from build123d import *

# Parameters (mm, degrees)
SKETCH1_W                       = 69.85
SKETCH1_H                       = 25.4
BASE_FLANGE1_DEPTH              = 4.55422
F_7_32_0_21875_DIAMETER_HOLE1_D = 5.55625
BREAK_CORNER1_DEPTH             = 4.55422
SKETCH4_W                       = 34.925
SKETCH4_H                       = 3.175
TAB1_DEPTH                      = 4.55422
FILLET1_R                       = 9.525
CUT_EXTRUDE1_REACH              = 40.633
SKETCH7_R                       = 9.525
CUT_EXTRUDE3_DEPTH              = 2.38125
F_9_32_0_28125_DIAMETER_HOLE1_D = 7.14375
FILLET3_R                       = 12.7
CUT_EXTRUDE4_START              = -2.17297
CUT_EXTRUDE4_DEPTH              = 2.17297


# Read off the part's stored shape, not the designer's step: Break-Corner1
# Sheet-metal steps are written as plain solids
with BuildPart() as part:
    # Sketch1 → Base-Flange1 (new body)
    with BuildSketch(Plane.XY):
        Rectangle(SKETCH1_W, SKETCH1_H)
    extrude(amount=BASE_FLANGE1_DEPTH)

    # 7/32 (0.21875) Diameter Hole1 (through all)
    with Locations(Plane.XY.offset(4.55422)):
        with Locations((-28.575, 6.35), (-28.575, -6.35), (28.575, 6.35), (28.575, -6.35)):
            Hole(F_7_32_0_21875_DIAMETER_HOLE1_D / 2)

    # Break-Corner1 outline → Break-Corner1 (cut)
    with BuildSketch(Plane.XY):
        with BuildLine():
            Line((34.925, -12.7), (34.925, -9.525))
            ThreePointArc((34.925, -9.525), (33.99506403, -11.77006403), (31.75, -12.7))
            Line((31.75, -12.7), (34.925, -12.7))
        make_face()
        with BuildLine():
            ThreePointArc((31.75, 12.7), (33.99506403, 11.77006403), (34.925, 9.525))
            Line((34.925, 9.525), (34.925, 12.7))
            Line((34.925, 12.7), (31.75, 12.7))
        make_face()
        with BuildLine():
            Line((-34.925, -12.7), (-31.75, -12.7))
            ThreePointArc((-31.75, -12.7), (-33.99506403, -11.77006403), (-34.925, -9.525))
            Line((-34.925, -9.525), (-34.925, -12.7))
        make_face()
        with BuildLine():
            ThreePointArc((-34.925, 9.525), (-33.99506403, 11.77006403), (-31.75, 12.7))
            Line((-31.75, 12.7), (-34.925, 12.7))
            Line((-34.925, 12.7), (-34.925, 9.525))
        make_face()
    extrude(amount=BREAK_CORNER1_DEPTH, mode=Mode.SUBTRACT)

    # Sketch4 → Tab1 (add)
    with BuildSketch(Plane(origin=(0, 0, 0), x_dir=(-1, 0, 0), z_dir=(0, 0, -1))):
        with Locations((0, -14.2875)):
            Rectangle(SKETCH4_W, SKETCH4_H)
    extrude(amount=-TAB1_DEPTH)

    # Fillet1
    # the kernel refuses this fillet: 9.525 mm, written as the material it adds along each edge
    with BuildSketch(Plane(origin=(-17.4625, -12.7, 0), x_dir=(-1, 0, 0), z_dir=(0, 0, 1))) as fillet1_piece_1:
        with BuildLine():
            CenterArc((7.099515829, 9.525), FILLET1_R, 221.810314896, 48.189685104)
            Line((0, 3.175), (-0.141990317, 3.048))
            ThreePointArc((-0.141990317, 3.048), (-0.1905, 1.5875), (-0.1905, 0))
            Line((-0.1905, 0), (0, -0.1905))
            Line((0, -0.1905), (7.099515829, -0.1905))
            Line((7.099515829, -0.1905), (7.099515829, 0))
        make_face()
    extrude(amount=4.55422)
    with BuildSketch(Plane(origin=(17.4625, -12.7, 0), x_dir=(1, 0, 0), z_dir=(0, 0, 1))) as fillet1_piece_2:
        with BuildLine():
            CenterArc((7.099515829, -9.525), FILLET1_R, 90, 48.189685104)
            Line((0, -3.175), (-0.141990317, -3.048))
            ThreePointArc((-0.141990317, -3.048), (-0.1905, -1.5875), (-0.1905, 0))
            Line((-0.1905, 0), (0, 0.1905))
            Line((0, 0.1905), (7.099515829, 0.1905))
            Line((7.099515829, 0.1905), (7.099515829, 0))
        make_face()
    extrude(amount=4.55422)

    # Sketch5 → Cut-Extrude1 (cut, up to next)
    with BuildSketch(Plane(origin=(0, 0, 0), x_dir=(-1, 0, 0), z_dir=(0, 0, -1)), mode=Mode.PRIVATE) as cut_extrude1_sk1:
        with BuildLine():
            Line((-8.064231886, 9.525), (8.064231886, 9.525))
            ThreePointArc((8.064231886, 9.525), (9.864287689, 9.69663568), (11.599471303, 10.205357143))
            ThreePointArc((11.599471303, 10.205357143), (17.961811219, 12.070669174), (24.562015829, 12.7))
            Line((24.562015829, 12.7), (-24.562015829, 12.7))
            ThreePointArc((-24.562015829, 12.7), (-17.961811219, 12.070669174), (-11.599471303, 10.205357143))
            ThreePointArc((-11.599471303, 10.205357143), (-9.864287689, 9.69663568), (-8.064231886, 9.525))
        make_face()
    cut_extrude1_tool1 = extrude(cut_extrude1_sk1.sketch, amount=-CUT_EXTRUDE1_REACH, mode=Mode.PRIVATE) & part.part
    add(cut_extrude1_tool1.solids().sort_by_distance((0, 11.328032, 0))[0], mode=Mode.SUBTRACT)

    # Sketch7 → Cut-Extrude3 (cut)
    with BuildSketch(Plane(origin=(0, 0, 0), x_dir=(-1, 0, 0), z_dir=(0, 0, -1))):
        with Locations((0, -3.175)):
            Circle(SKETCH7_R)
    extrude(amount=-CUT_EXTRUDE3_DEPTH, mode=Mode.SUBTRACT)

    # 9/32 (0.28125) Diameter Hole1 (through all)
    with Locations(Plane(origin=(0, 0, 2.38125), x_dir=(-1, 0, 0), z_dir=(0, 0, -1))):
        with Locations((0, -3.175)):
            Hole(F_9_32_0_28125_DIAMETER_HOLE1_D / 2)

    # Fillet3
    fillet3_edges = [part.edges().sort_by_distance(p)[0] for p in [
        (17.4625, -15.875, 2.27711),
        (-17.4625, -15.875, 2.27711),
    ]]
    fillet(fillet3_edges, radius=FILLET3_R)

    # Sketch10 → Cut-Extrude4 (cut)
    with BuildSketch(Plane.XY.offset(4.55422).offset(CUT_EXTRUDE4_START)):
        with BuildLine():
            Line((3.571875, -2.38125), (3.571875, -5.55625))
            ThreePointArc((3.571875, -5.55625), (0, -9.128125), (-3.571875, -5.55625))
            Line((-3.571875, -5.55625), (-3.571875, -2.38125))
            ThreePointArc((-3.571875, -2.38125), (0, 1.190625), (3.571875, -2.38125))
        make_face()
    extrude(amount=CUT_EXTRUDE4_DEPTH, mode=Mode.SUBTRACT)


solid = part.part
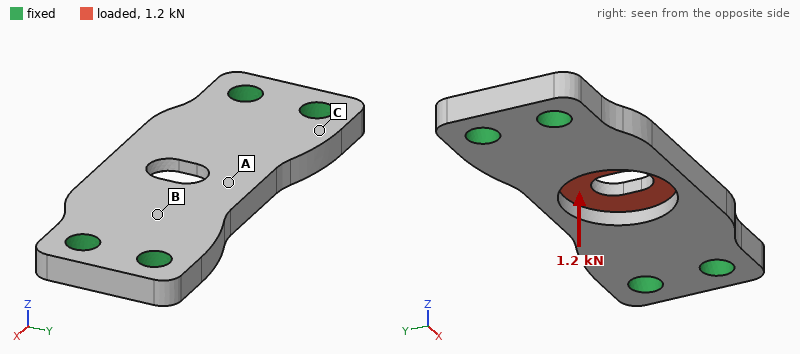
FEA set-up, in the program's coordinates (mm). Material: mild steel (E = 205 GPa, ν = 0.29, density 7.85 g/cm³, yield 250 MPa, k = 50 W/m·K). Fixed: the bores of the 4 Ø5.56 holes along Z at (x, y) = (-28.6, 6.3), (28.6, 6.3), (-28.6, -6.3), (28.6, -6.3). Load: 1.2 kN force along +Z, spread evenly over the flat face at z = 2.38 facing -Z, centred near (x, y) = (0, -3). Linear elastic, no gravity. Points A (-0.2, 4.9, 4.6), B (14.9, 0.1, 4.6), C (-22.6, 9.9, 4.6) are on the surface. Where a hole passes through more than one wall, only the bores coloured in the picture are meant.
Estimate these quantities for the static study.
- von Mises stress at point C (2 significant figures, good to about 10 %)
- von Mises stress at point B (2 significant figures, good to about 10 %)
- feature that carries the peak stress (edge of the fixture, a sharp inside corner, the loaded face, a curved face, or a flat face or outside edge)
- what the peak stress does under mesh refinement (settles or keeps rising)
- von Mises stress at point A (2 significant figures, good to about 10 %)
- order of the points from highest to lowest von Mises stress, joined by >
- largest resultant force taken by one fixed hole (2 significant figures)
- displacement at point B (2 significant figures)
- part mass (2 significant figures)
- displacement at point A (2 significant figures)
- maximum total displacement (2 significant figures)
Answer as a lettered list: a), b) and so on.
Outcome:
a) 57 MPa
b) 23 MPa
c) edge of the fixture
d) keeps rising
e) 110 MPa
f) A > C > B
g) 490 N
h) 13 µm
i) 54 g
j) 31 µm
k) 36 µm
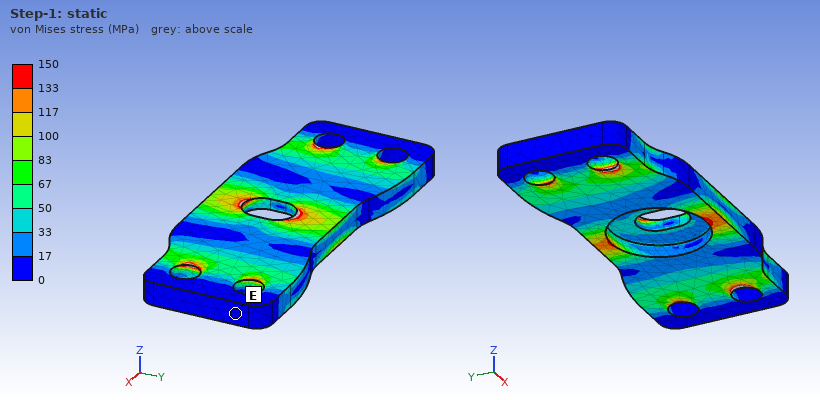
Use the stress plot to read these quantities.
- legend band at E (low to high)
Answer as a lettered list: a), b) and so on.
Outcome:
a) 0 to 17 MPa
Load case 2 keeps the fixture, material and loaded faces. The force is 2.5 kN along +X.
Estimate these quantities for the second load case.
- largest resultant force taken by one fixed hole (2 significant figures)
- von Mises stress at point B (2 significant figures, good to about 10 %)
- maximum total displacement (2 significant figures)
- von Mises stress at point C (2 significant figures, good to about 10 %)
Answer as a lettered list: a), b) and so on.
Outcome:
a) 730 N
b) 18 MPa
c) 2.4 µm
d) 8.8 MPa
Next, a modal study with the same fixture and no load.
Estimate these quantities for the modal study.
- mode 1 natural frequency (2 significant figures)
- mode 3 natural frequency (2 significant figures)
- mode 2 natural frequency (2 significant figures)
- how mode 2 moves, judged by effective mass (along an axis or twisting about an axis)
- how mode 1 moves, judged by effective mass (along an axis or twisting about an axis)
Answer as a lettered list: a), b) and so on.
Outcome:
a) 8100 Hz
b) 18 kHz
c) 12 kHz
d) twisting about X
e) along Z
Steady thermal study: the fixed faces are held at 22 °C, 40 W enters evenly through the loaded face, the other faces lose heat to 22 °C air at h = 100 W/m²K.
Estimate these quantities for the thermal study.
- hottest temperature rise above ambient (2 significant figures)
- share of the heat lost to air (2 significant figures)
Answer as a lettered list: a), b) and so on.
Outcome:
a) 80 K
b) 27 %
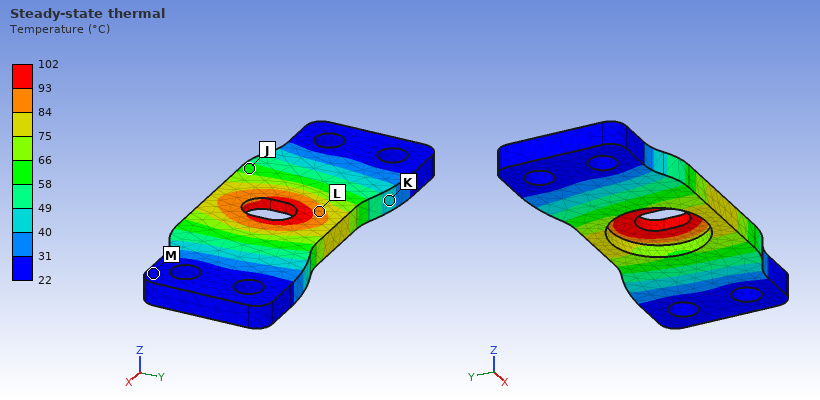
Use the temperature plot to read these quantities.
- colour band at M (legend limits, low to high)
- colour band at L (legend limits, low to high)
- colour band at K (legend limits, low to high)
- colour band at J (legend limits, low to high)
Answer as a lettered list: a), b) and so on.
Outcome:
a) 22 to 31 °C
b) 84 to 93 °C
c) 40 to 49 °C
d) 58 to 66 °C
